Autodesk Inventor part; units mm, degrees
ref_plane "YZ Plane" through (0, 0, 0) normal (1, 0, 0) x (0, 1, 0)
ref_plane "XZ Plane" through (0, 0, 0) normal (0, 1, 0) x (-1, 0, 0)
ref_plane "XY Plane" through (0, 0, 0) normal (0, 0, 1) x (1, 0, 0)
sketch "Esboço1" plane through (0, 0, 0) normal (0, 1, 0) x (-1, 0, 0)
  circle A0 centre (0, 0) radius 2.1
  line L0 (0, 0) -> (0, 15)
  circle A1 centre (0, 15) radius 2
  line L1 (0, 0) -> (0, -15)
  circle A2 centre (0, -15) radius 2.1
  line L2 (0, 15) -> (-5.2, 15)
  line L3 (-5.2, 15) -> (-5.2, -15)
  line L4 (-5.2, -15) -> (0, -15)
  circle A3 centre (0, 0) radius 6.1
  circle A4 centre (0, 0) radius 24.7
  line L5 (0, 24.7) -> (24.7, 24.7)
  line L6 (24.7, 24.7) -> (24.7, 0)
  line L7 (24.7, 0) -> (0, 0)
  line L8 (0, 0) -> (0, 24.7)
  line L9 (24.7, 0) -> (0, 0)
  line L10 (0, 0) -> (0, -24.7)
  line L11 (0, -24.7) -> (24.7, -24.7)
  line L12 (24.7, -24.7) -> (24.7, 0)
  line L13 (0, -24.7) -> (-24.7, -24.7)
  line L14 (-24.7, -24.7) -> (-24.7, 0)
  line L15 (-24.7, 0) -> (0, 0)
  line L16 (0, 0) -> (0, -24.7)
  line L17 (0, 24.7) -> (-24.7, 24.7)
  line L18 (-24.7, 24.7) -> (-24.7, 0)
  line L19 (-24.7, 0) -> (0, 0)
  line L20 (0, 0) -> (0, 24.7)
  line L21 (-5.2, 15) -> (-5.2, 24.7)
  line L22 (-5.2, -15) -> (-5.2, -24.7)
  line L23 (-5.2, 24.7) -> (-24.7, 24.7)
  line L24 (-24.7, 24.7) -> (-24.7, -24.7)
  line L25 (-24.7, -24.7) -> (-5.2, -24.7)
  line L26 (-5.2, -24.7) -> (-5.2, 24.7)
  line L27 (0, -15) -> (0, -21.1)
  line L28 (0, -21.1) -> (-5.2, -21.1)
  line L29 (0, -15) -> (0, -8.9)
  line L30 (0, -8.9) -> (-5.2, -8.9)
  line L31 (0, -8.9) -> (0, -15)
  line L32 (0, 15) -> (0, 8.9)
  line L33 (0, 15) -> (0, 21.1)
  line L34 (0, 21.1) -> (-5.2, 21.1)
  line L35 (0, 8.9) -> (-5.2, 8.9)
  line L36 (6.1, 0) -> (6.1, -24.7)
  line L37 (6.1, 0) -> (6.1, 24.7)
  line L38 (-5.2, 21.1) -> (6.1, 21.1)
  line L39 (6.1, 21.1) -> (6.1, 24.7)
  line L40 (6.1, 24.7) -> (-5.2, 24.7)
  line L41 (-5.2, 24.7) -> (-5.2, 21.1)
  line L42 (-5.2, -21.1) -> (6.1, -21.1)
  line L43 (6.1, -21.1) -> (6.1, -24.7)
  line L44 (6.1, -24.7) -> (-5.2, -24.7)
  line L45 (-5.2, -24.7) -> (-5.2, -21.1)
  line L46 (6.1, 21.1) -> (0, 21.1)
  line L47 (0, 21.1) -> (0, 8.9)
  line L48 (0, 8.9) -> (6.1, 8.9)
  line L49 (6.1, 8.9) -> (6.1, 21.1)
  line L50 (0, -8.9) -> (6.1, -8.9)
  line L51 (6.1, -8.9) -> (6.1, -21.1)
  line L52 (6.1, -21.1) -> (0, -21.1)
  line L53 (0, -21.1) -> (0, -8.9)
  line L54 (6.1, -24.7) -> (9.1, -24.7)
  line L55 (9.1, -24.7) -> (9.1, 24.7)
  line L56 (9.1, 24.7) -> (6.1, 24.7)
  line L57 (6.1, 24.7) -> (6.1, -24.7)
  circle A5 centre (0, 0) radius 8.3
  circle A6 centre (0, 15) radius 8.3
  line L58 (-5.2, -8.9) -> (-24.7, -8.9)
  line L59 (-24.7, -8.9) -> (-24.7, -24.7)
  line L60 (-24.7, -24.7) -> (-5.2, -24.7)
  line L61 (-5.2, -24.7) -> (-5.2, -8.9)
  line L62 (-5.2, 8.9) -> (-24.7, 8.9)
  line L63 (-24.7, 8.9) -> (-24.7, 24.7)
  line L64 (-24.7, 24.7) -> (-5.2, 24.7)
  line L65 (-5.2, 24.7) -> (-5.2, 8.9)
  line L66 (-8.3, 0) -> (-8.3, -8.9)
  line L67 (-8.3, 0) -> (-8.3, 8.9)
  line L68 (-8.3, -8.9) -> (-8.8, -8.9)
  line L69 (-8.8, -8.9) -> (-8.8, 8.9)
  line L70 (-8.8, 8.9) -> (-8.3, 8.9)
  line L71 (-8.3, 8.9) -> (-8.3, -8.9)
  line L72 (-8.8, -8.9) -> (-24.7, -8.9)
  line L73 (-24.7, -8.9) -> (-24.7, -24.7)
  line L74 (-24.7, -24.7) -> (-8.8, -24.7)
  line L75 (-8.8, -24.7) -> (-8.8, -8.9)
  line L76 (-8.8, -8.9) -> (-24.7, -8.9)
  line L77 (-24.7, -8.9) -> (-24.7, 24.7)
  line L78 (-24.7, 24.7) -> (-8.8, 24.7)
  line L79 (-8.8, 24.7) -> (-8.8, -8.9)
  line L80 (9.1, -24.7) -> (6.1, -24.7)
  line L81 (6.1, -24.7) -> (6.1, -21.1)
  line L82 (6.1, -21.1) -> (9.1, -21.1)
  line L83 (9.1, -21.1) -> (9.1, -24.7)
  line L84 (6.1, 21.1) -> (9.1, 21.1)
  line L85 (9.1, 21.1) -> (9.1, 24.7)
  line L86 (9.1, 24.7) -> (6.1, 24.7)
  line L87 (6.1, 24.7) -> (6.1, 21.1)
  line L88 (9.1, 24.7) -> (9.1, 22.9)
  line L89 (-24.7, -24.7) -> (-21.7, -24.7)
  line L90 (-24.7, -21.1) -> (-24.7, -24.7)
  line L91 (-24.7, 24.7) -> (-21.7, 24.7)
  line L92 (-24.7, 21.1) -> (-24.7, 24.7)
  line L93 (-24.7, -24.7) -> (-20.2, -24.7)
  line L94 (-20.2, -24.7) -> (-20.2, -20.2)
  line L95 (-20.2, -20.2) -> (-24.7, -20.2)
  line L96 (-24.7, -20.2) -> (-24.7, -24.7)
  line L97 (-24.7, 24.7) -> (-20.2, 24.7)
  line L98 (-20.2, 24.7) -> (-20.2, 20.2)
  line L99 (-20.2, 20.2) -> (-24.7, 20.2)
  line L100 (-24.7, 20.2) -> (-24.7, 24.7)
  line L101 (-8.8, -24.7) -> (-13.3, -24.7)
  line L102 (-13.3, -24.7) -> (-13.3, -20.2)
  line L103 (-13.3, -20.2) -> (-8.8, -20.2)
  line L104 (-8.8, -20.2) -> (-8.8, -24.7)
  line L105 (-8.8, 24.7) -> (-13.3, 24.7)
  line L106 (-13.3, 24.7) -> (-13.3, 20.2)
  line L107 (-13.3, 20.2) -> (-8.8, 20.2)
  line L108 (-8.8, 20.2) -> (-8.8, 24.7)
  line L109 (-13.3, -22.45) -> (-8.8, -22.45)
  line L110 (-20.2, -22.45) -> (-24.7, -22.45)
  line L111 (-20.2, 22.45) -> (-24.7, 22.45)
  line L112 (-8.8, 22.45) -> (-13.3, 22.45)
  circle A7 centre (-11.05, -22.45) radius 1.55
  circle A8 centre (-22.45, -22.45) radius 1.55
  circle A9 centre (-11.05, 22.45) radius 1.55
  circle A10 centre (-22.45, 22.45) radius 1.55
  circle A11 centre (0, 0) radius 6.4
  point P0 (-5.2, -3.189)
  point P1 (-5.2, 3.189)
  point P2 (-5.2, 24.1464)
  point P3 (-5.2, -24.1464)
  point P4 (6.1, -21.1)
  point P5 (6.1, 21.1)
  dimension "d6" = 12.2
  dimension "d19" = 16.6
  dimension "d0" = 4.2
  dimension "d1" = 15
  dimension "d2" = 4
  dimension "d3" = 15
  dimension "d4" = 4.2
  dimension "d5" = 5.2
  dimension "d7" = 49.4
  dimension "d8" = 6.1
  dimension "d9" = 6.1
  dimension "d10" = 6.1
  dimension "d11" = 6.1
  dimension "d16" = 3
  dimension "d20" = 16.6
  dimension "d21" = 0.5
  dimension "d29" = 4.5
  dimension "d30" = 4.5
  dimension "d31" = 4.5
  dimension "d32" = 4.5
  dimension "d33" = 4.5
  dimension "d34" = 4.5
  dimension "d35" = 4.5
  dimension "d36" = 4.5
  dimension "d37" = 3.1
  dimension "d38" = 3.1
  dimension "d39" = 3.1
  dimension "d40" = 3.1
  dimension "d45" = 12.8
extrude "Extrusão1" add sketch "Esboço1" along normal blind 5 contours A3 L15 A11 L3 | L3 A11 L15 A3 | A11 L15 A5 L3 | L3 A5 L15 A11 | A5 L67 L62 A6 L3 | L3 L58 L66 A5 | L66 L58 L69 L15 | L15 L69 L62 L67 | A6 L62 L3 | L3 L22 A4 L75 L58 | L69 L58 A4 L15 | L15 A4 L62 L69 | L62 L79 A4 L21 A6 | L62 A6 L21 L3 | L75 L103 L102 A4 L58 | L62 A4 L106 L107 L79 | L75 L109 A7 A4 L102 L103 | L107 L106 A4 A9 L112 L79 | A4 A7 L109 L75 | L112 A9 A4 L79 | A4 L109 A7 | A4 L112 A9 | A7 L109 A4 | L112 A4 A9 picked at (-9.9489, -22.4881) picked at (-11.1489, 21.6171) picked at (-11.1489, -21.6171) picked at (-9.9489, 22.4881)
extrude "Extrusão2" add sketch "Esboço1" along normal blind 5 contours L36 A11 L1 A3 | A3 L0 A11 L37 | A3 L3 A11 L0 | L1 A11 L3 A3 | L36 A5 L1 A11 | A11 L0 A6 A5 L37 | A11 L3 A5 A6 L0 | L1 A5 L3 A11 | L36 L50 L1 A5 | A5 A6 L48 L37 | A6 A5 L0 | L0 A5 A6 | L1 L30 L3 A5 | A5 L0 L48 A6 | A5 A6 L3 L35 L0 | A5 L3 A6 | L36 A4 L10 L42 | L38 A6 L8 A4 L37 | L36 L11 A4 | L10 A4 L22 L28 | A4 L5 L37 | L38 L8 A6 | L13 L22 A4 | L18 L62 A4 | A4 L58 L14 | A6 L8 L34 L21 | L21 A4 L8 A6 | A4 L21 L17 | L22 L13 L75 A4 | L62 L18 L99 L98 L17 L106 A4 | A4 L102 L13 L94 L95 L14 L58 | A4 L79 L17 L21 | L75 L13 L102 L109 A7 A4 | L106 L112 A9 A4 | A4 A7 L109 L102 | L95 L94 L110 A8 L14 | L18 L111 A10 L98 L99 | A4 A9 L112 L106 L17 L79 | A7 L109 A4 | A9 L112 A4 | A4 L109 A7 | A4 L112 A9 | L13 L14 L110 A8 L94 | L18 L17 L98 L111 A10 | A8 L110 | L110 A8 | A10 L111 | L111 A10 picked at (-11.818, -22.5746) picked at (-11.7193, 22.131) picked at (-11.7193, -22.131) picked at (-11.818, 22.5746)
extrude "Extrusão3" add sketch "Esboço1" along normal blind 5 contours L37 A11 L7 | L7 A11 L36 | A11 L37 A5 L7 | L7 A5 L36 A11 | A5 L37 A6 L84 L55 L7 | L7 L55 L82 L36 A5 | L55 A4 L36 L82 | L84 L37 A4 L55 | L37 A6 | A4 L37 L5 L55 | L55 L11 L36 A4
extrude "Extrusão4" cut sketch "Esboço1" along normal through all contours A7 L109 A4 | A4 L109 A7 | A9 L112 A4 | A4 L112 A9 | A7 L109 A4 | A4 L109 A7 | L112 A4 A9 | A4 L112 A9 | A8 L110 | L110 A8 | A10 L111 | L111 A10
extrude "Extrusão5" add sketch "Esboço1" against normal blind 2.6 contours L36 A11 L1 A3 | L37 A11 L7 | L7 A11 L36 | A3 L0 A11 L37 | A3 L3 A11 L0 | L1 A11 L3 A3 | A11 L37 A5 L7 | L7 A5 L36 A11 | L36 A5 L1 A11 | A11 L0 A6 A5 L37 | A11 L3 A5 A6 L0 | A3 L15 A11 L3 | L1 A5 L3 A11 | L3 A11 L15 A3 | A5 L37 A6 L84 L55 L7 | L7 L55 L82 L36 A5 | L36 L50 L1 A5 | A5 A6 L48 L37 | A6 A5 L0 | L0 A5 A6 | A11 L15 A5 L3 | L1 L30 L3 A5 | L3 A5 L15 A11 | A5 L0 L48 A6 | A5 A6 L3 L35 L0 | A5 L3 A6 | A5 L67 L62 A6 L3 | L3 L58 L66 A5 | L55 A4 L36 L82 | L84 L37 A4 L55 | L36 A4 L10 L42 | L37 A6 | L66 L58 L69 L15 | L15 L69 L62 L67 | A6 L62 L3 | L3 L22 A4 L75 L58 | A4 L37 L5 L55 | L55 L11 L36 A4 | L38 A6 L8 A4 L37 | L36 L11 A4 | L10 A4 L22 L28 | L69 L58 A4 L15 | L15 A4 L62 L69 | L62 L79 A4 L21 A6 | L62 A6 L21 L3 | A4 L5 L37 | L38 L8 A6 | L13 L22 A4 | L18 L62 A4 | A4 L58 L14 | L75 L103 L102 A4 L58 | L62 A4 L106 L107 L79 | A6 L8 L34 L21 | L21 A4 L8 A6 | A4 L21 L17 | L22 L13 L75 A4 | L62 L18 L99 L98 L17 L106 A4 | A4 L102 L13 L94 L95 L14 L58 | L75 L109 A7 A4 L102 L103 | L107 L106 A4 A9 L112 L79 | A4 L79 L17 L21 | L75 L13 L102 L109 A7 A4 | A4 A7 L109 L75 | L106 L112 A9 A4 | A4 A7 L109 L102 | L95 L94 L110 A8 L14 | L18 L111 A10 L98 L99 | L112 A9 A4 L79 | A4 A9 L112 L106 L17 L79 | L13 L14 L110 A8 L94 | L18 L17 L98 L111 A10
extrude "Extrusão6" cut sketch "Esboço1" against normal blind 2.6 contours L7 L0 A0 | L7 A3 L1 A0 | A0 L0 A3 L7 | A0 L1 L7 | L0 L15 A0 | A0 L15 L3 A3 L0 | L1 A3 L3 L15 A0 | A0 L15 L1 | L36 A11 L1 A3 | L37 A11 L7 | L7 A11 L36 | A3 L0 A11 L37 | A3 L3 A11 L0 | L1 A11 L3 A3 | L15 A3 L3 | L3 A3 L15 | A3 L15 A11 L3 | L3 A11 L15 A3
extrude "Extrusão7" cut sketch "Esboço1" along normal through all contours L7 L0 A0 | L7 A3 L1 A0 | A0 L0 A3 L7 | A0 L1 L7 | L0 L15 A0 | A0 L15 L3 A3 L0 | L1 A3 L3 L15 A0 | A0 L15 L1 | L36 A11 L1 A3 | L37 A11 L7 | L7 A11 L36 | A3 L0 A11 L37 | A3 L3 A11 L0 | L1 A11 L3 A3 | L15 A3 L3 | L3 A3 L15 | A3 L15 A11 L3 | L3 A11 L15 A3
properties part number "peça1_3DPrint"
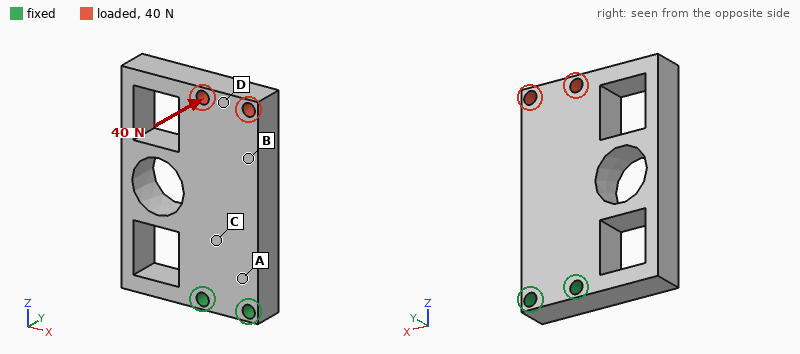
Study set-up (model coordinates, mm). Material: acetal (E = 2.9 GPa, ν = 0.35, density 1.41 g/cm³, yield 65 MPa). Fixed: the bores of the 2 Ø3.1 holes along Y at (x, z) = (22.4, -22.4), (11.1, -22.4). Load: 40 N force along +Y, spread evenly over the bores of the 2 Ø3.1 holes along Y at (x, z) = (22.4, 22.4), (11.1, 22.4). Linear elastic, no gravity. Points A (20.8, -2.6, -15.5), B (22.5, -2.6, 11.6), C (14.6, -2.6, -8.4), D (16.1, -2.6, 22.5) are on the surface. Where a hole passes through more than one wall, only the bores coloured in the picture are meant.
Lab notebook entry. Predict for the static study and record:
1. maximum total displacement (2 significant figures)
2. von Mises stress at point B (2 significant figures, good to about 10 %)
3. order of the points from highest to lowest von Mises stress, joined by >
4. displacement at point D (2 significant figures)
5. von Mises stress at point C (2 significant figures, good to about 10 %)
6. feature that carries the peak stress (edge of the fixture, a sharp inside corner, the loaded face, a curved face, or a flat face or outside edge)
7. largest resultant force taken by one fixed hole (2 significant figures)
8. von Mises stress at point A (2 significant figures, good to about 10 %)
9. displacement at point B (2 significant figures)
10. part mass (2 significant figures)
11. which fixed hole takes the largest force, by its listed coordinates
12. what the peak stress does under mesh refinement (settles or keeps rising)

0.62 mm
2.2 MPa
A > C > B > D
0.57 mm
5.7 MPa
edge of the fixture
25 N
8.0 MPa
0.38 mm
13 g
(11.1, -22.4)
keeps rising
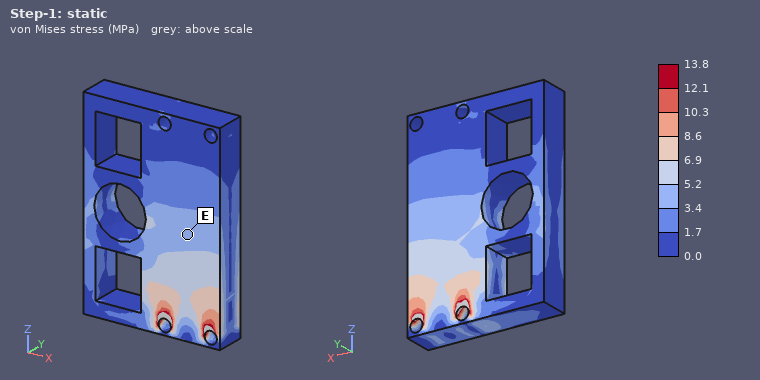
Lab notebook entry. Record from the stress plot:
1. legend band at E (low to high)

3.4 to 5.2 MPa
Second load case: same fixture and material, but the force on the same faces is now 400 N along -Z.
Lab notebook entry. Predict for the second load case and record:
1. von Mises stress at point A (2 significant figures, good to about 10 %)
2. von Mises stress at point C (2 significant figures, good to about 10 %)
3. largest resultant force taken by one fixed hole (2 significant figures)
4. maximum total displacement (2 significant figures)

3.5 MPa
2.7 MPa
210 N
94 µm
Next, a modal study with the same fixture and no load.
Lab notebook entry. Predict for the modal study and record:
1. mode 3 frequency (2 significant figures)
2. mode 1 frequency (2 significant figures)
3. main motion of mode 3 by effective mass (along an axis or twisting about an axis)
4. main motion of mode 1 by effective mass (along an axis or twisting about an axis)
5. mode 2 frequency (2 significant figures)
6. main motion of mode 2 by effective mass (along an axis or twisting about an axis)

1700 Hz
680 Hz
twisting about Z
along Y
1400 Hz
along X
